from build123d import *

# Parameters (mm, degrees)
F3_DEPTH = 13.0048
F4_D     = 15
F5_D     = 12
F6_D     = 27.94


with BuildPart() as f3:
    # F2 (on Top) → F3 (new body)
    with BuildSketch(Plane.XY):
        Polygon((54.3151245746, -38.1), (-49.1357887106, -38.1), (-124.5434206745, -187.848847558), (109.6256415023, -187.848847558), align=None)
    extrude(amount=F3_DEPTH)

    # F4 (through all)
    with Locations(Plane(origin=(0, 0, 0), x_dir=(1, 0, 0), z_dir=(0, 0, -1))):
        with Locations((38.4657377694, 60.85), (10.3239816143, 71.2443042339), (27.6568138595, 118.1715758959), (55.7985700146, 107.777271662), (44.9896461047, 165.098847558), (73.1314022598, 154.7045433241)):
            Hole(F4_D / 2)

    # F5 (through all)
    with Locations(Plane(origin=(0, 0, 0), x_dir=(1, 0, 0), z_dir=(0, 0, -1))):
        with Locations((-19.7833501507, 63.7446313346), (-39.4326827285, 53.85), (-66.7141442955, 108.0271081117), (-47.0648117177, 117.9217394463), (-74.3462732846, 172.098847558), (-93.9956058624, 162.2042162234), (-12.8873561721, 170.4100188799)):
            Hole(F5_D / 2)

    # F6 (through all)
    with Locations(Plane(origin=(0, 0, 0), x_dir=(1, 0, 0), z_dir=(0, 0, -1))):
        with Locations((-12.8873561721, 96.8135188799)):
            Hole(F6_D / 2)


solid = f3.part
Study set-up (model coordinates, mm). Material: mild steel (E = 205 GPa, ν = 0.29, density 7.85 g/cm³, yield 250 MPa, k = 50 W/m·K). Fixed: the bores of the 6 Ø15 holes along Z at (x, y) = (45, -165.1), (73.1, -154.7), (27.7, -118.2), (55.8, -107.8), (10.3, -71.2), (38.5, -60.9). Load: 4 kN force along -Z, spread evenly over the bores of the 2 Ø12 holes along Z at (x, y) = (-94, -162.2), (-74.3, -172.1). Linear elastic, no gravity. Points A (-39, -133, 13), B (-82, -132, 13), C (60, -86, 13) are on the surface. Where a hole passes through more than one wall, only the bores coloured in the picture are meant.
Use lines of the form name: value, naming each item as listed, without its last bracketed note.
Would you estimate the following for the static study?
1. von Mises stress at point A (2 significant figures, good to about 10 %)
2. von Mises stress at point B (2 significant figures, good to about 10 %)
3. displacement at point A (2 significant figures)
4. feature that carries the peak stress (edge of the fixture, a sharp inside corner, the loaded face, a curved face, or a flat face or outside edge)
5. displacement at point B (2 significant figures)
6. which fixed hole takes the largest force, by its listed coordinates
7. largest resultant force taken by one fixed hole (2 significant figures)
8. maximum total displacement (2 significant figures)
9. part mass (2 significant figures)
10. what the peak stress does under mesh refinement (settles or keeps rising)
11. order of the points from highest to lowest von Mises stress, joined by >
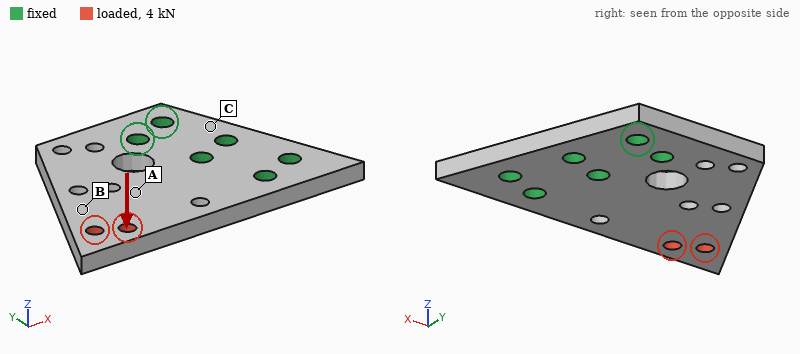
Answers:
von Mises stress at point A: 76 MPa
von Mises stress at point B: 47 MPa
displacement at point A: 0.19 mm
feature that carries the peak stress: edge of the fixture
displacement at point B: 0.41 mm
which fixed hole takes the largest force, by its listed coordinates: (27.7, -118.2)
largest resultant force taken by one fixed hole: 3.6 kN
maximum total displacement: 0.86 mm
part mass: 2.3 kg
what the peak stress does under mesh refinement: keeps rising
order of the points from highest to lowest von Mises stress, joined by >: A > B > C
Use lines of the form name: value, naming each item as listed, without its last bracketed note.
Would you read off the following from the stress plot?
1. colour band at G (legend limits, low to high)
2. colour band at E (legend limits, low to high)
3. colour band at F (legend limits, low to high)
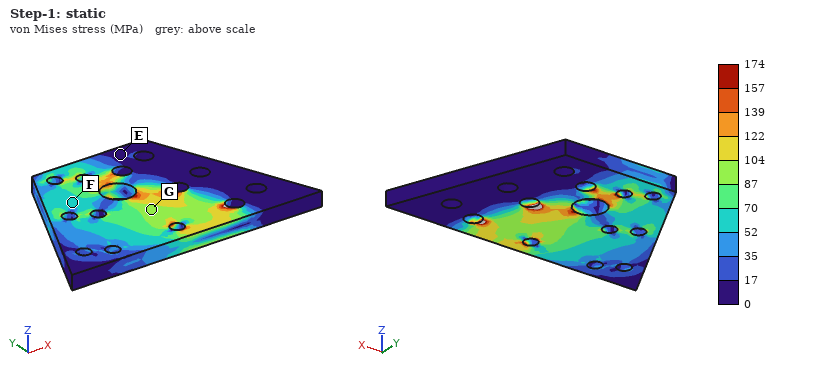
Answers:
colour band at G: 87 to 104 MPa
colour band at E: 0 to 17 MPa
colour band at F: 52 to 70 MPa
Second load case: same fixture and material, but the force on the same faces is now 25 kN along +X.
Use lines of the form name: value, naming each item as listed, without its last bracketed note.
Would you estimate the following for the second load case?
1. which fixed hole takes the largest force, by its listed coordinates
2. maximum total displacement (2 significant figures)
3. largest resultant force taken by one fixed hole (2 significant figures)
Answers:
which fixed hole takes the largest force, by its listed coordinates: (45, -165.1)
maximum total displacement: 44 µm
largest resultant force taken by one fixed hole: 16 kN
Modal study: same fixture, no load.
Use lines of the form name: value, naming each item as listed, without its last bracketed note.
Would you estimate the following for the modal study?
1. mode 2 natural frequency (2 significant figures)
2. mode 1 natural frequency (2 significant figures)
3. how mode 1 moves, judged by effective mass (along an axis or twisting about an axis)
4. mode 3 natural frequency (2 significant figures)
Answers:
mode 2 natural frequency: 2100 Hz
mode 1 natural frequency: 690 Hz
how mode 1 moves, judged by effective mass: along Z
mode 3 natural frequency: 3200 Hz
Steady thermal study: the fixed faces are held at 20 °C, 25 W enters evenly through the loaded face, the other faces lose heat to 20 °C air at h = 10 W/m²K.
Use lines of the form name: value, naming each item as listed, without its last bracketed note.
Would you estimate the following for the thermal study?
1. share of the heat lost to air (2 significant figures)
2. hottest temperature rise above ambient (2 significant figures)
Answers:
share of the heat lost to air: 26 %
hottest temperature rise above ambient: 48 K
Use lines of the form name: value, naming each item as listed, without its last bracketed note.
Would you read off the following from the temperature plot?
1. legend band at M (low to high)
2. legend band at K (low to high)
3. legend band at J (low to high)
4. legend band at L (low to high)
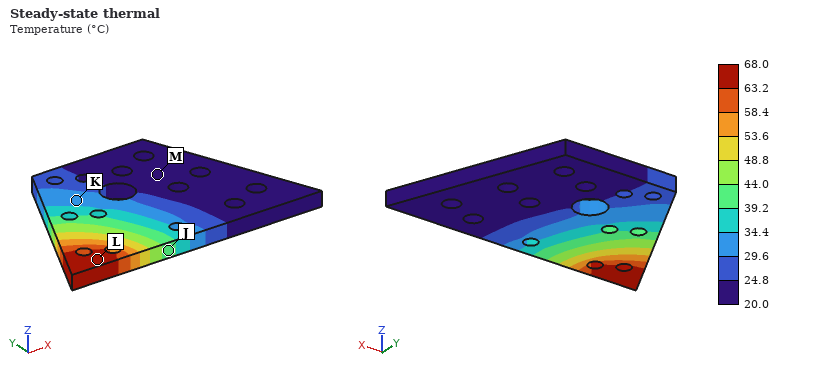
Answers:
legend band at M: 20.0 to 24.8 °C
legend band at K: 29.6 to 34.4 °C
legend band at J: 39.2 to 44.0 °C
legend band at L: 63.2 to 68.0 °C
